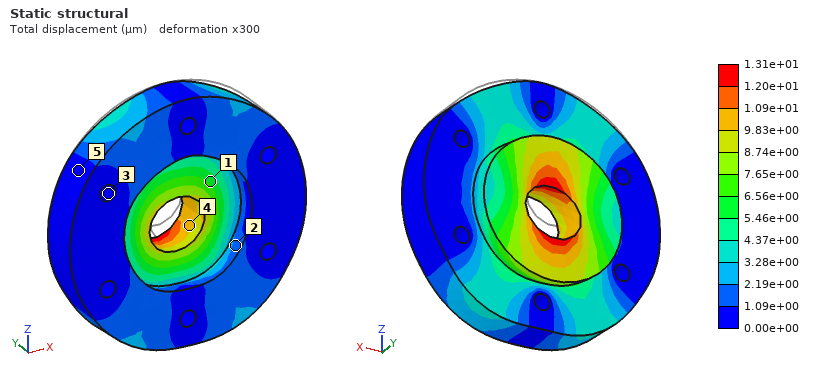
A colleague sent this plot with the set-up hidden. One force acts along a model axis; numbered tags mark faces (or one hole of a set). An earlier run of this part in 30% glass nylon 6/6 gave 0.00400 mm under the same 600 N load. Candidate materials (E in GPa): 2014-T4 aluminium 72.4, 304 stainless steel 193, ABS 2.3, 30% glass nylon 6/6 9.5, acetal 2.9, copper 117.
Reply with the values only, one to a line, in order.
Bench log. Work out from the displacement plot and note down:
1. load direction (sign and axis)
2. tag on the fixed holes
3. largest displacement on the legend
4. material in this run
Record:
-Z
3
1.31e+01 µm
acetal
